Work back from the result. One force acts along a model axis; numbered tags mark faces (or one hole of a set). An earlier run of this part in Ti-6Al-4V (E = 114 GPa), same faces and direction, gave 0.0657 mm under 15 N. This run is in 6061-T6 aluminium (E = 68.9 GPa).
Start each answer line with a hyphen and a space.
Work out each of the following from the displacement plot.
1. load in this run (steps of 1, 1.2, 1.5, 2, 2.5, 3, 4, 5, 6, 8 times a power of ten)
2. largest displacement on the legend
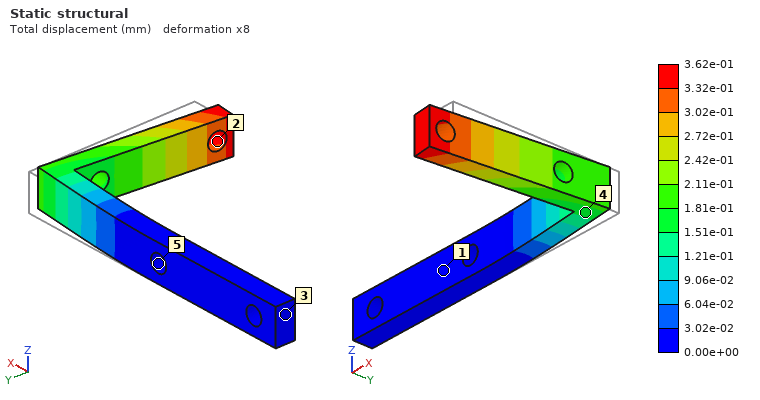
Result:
- 50 N
- 3.62e-01 mm
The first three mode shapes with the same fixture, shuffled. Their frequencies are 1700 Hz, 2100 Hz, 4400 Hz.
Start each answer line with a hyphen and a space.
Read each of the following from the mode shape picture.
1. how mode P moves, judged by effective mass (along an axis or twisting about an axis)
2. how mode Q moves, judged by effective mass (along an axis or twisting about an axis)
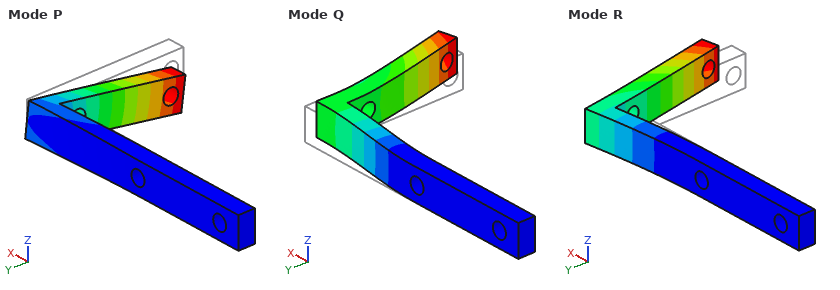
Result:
- along Z
- along Y
